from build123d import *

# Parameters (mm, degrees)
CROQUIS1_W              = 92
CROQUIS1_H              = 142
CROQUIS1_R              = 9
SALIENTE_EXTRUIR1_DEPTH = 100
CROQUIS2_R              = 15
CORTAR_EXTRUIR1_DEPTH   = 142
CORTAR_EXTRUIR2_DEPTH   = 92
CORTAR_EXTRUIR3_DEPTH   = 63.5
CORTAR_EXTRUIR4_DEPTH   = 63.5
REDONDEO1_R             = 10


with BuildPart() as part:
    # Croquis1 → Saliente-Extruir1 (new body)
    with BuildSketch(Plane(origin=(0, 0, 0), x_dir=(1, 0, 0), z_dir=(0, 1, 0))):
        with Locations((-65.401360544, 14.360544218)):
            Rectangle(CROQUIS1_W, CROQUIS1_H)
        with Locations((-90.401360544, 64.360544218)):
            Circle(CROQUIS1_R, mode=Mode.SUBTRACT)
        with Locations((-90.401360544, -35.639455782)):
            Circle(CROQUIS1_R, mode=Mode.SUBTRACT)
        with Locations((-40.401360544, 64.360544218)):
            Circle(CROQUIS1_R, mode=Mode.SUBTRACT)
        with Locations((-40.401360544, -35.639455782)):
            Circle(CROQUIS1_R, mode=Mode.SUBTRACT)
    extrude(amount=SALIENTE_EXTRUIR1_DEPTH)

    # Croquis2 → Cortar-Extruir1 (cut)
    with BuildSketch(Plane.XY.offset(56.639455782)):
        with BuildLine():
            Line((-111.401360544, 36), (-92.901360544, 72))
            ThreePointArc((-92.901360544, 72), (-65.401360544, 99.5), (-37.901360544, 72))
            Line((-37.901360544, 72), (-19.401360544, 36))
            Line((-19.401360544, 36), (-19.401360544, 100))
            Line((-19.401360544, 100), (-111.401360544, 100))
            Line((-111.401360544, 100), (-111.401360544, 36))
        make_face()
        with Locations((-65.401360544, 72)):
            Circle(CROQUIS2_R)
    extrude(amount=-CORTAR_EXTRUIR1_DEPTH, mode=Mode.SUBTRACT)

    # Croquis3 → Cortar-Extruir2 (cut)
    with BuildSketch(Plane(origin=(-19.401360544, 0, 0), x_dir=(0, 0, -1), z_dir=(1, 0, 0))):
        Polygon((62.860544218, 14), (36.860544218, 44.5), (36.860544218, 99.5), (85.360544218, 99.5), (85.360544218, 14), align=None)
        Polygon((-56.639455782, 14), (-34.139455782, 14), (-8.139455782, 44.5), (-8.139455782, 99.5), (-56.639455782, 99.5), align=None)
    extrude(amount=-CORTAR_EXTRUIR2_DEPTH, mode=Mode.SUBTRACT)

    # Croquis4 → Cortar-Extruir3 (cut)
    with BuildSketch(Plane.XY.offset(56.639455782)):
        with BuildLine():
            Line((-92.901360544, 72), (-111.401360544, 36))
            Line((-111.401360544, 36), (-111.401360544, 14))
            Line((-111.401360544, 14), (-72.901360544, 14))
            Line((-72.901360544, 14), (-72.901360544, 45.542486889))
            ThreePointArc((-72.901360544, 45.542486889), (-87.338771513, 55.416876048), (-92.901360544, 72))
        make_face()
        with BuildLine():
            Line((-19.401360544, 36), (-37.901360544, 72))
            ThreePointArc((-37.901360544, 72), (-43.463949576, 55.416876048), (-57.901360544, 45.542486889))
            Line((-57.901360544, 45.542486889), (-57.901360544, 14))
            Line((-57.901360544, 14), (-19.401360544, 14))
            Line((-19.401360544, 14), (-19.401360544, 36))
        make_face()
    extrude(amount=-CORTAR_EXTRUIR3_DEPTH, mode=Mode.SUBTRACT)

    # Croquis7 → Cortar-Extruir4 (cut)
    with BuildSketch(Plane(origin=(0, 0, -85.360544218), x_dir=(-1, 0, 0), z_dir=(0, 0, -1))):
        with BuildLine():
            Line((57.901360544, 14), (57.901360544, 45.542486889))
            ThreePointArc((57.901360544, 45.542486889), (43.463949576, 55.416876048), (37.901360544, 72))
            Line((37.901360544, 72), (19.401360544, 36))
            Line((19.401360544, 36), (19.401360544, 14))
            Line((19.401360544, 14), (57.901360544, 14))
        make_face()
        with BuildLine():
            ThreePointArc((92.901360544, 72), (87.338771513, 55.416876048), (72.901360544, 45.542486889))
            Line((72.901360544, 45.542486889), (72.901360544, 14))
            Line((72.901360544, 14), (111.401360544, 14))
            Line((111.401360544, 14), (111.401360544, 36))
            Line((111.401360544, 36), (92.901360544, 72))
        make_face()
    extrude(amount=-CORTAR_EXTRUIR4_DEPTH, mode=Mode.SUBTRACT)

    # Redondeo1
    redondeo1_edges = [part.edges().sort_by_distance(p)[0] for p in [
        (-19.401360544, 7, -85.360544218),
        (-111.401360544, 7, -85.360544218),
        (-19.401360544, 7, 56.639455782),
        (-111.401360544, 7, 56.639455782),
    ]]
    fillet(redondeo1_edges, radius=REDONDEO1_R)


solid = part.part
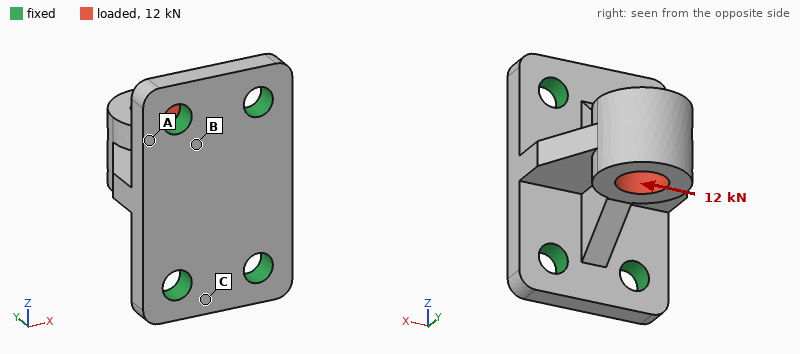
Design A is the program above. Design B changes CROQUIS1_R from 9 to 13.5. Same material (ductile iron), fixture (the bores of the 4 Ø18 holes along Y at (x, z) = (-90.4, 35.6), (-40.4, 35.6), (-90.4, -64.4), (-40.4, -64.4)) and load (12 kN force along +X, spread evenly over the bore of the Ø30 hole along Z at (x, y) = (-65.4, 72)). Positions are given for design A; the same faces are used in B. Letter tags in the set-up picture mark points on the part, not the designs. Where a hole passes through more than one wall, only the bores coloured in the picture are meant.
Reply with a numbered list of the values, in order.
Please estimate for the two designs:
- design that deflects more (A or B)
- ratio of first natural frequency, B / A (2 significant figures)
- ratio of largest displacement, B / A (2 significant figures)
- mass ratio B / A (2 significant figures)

1. A
2. 1.1
3. 0.81
4. 0.94
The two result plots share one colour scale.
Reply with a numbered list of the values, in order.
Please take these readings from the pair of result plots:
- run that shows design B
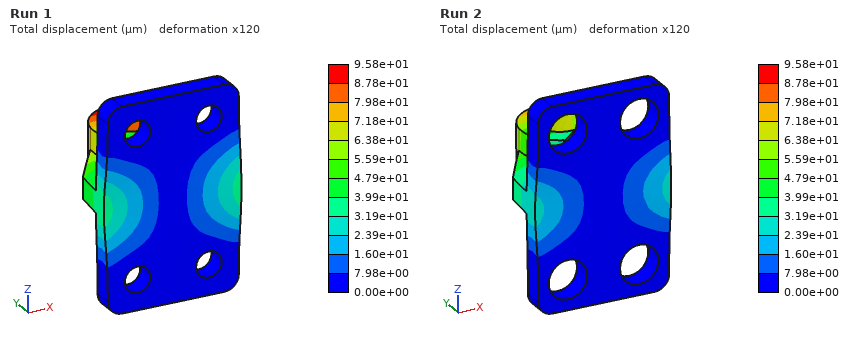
1. Run 2
